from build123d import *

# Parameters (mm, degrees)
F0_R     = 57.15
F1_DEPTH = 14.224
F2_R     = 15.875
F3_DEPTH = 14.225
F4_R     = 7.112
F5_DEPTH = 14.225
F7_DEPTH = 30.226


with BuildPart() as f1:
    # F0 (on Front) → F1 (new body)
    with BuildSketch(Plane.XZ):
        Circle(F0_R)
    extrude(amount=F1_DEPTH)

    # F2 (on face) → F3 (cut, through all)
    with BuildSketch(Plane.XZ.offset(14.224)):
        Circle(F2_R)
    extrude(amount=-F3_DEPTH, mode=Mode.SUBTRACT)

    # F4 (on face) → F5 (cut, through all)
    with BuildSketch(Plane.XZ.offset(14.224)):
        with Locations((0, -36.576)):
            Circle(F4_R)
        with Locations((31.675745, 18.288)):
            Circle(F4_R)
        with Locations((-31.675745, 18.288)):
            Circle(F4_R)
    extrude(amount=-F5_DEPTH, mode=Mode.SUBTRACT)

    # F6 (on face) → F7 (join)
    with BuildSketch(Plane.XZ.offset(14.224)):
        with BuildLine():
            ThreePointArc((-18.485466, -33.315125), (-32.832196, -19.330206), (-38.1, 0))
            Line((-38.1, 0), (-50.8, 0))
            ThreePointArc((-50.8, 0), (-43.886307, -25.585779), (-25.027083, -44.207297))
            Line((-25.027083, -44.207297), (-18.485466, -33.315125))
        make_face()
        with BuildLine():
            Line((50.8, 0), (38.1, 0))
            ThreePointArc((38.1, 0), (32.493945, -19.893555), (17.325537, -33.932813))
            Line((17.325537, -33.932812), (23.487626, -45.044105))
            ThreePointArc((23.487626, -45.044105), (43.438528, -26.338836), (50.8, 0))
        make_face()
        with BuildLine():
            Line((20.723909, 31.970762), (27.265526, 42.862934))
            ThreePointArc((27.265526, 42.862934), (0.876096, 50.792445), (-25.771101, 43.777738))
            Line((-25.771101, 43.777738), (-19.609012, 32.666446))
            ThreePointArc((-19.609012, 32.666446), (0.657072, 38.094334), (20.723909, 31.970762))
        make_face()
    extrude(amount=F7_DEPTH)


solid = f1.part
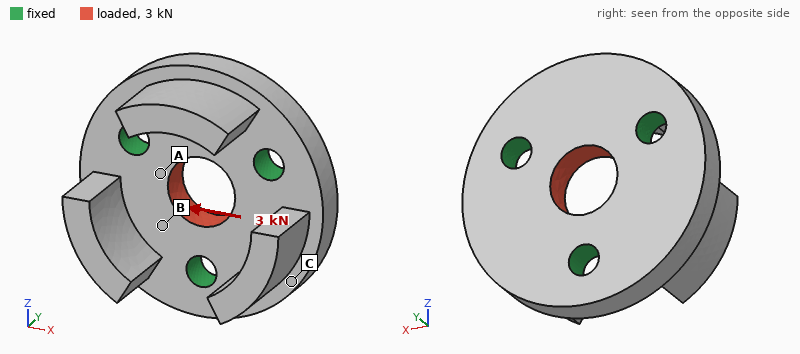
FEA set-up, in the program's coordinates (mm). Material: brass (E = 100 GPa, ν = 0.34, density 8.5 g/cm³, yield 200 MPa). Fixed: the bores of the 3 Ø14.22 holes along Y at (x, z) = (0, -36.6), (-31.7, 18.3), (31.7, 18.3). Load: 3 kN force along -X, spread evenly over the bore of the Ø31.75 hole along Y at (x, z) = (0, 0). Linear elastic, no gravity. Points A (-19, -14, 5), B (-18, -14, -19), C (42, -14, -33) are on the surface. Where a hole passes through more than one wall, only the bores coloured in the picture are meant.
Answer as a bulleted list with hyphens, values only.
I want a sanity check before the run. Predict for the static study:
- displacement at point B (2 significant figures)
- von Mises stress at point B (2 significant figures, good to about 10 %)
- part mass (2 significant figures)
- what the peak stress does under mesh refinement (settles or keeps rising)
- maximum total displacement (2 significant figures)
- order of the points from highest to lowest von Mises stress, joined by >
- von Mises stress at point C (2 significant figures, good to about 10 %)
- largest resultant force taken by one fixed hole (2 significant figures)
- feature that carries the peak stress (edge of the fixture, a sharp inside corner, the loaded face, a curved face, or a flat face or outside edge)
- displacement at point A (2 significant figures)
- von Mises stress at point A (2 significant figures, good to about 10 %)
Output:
- 0.57 µm
- 1.5 MPa
- 1.6 kg
- keeps rising
- 0.84 µm
- A > B > C
- 0.66 MPa
- 1.0 kN
- edge of the fixture
- 0.49 µm
- 2.3 MPa
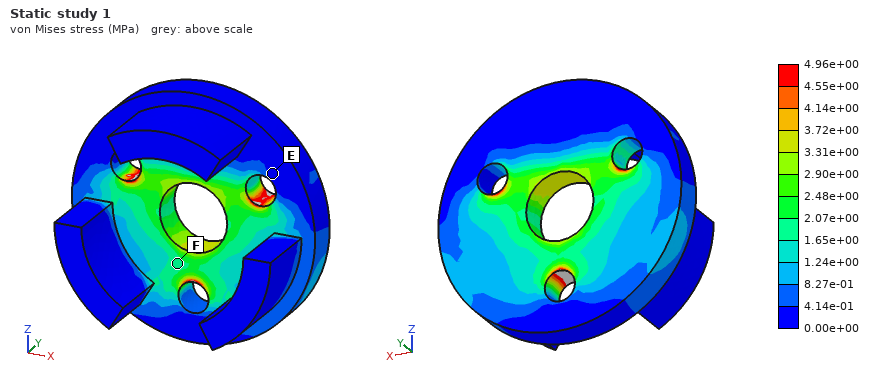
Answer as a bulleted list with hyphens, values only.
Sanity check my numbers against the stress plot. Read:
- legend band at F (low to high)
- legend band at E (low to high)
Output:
- 1.65e+00 to 2.07e+00 MPa
- 0.00e+00 to 4.14e-01 MPa
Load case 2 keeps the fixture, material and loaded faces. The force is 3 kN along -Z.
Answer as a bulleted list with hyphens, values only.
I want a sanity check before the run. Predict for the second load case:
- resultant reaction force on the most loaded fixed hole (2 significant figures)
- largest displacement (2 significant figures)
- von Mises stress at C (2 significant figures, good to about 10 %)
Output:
- 1.0 kN
- 0.91 µm
- 0.44 MPa
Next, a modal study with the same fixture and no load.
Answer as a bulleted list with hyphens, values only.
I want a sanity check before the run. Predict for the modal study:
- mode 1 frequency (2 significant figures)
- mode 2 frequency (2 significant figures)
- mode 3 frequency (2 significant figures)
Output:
- 3200 Hz
- 3200 Hz
- 3200 Hz
